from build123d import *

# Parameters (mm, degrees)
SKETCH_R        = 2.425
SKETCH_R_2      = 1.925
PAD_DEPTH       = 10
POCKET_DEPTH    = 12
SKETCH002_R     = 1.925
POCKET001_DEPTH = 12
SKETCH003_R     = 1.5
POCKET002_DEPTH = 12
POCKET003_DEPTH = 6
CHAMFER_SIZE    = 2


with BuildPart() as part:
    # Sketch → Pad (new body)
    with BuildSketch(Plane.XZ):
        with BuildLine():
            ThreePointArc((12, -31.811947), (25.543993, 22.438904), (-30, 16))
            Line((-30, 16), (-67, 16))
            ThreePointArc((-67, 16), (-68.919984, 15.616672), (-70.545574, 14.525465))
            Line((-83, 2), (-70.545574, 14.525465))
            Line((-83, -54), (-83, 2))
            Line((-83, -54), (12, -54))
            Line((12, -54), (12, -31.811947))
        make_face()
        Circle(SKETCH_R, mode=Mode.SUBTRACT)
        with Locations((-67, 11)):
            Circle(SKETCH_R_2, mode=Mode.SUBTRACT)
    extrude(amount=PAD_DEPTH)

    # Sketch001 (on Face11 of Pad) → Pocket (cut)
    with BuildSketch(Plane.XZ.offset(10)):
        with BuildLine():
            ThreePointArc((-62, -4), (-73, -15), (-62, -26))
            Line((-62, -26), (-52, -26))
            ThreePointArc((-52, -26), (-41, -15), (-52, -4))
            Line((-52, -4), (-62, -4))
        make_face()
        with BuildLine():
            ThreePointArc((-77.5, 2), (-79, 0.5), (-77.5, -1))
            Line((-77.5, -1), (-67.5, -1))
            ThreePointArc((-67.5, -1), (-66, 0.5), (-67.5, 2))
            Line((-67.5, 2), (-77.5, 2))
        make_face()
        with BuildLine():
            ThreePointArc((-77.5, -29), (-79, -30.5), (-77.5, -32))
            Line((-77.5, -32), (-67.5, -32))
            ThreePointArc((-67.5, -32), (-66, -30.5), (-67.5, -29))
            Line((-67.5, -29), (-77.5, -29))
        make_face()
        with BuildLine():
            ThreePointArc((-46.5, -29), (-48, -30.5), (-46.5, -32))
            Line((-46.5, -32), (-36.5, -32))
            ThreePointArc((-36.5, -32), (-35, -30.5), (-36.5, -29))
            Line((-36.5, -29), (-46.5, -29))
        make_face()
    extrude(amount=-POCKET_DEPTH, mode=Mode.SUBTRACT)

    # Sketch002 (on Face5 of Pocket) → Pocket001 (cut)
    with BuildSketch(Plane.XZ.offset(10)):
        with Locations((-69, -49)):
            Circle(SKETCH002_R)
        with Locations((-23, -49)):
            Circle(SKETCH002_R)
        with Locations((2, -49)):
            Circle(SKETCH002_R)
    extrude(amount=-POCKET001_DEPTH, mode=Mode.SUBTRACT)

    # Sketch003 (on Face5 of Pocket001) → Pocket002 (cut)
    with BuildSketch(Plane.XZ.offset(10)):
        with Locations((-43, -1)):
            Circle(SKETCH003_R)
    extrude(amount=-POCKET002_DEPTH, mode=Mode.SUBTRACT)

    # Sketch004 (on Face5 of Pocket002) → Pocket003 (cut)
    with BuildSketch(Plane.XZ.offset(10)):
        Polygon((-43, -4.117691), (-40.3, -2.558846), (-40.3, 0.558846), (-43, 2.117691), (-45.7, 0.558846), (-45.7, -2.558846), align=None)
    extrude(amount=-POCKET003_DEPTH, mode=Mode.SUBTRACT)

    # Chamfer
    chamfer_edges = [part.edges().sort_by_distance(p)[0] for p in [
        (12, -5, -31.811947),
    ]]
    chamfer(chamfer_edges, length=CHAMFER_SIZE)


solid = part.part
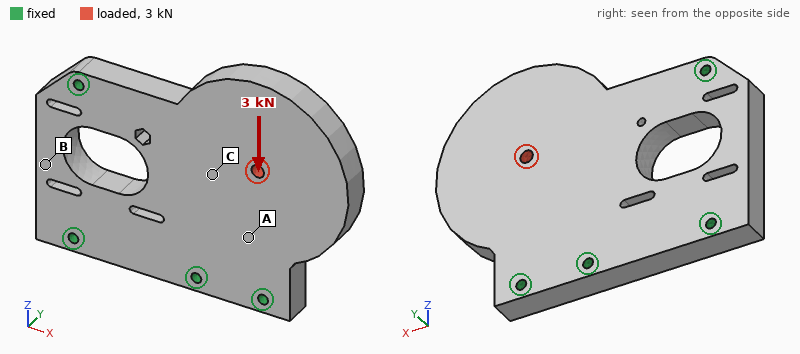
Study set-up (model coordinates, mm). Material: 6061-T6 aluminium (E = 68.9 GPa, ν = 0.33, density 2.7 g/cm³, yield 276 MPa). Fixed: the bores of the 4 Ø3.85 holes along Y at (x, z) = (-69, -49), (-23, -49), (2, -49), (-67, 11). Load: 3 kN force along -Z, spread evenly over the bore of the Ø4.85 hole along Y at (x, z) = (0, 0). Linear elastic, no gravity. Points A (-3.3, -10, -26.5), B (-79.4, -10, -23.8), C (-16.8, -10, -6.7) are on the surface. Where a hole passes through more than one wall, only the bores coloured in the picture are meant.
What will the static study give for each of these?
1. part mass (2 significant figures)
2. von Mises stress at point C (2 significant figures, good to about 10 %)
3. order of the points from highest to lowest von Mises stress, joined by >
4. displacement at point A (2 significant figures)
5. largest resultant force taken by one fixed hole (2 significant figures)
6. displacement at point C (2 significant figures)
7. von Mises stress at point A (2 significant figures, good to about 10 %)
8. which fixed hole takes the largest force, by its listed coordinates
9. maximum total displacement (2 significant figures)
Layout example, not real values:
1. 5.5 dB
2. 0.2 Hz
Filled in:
1. 200 g
2. 4.5 MPa
3. A > C > B
4. 3.1 µm
5. 1.8 kN
6. 3.4 µm
7. 7.7 MPa
8. (2, -49)
9. 8.4 µm
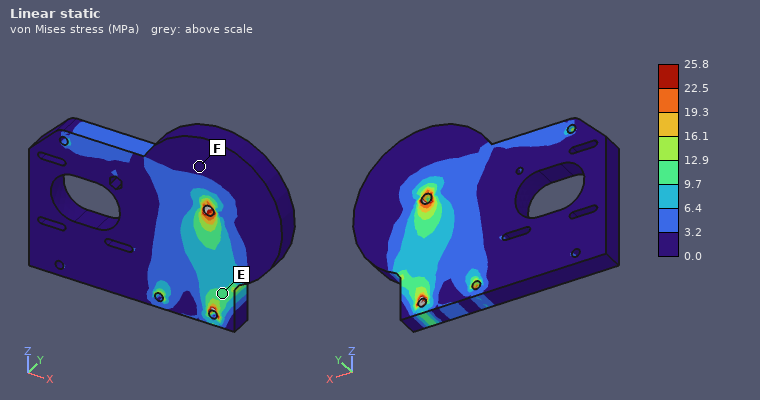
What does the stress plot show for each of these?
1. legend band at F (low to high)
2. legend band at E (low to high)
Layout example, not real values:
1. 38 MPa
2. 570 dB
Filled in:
1. 0.0 to 3.2 MPa
2. 9.7 to 12.9 MPa
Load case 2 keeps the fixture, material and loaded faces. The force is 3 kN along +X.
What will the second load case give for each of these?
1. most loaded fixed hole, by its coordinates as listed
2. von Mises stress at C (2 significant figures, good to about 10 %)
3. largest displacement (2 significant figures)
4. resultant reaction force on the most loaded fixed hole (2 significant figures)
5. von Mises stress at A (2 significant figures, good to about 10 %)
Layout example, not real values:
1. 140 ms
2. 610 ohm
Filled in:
1. (-67, 11)
2. 6.6 MPa
3. 11 µm
4. 1.8 kN
5. 4.1 MPa
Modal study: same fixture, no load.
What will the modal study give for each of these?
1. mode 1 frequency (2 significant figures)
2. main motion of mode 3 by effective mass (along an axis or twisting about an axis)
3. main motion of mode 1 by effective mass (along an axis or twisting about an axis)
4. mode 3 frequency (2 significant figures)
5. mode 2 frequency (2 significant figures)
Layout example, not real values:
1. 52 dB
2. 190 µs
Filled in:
1. 1500 Hz
2. along Y
3. along Y
4. 7000 Hz
5. 4800 Hz
